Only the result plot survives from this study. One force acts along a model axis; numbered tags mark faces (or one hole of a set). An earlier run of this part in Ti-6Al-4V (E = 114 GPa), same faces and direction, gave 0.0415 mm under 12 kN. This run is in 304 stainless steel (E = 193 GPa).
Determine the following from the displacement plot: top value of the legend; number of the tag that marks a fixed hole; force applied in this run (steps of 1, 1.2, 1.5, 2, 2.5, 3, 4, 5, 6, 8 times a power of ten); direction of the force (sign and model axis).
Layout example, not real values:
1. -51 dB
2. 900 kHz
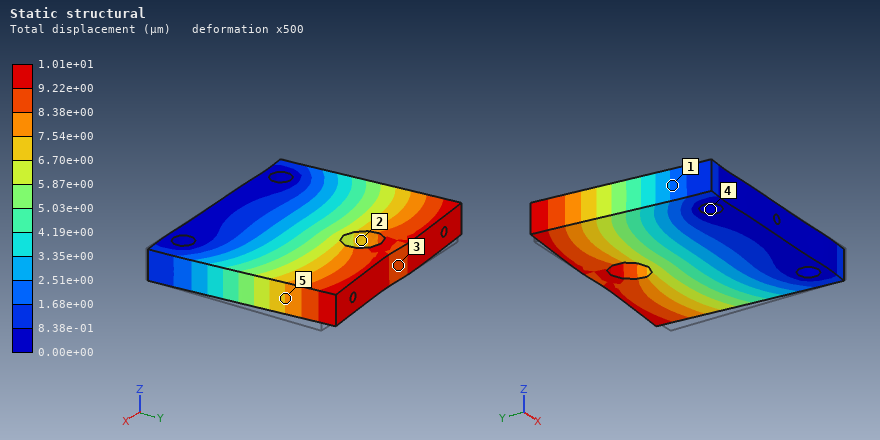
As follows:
1. 1.01e+01 µm
2. 4
3. 5 kN
4. -X
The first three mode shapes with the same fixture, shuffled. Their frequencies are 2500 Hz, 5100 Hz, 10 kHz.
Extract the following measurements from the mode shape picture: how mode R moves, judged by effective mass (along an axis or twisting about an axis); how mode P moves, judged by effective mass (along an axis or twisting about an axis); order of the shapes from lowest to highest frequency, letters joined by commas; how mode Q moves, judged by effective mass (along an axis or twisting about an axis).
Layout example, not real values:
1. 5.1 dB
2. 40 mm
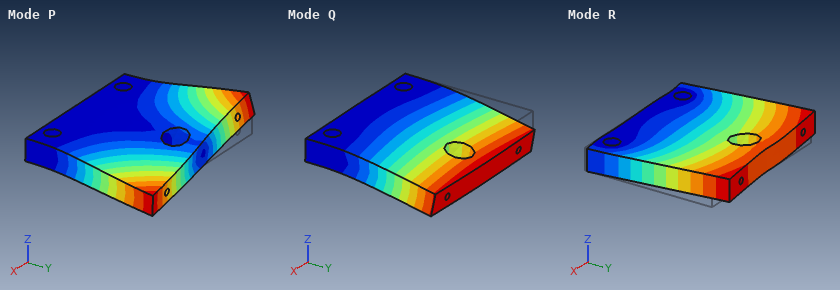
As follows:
1. along X
2. twisting about Y
3. Q, P, R
4. along Z
